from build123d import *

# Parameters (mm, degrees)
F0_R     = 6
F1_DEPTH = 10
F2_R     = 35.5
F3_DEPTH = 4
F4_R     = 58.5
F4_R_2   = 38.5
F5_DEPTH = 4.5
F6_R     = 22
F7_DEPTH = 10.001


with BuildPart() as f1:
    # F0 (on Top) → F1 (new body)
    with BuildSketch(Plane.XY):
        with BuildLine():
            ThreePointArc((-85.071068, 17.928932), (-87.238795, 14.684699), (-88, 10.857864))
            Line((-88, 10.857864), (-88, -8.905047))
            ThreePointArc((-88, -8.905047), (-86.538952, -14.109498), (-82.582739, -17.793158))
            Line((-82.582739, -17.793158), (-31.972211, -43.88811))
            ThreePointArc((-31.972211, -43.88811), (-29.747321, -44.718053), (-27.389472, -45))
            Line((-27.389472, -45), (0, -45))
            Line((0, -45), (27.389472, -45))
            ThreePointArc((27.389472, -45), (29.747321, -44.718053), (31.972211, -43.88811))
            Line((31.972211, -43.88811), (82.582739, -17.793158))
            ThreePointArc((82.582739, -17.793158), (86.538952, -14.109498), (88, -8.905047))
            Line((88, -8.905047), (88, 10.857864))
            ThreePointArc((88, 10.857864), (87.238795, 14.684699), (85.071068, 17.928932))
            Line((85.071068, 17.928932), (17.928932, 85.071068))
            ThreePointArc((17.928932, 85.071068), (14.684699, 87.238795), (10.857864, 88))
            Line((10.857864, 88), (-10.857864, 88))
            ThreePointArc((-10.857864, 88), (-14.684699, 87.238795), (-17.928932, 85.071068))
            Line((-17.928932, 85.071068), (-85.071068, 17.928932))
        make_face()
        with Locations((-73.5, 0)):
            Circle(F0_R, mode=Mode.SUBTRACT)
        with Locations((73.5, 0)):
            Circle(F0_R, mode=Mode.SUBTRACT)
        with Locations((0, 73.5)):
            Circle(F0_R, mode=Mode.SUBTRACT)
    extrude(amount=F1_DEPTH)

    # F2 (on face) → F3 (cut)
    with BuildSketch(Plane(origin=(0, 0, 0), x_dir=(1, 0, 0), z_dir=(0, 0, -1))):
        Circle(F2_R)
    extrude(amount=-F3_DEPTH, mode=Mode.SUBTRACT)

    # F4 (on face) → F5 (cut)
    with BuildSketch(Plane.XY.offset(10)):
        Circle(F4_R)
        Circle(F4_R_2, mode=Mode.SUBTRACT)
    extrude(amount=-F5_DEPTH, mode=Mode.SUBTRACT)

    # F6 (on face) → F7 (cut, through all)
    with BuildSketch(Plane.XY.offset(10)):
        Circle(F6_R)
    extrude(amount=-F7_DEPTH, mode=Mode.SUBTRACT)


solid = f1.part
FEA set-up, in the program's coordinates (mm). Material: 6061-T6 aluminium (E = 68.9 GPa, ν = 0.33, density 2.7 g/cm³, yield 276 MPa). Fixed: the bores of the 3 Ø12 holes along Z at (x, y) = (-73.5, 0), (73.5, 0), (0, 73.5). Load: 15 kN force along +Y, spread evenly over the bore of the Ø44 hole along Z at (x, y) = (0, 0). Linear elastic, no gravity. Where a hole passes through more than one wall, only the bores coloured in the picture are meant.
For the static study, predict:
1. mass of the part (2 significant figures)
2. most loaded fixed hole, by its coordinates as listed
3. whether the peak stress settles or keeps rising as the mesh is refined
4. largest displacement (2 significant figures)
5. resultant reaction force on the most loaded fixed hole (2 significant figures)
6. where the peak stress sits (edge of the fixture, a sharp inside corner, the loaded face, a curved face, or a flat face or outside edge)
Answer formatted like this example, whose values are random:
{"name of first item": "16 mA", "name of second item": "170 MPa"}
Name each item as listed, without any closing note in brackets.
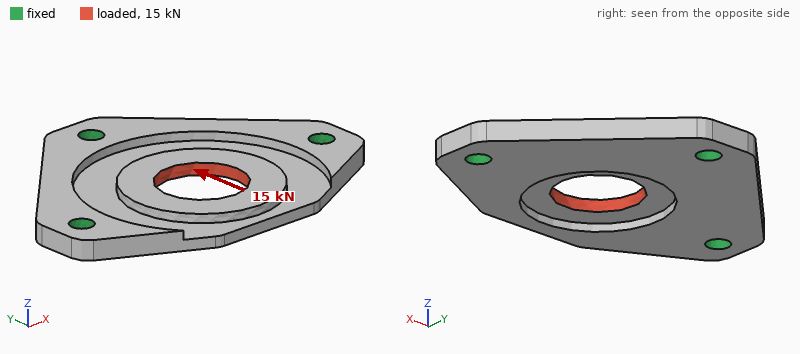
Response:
{"mass of the part": "300 g", "most loaded fixed hole, by its coordinates as listed": "(0, 73.5)", "whether the peak stress settles or keeps rising as the mesh is refined": "keeps rising", "largest displacement": "0.15 mm", "resultant reaction force on the most loaded fixed hole": "6.6 kN", "where the peak stress sits": "a sharp inside corner"}
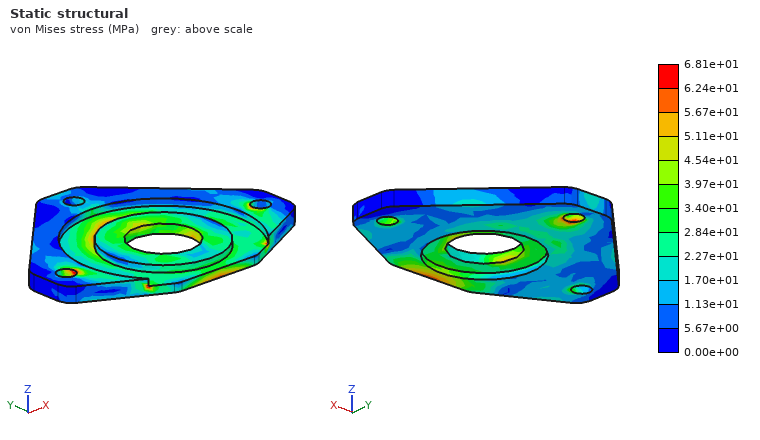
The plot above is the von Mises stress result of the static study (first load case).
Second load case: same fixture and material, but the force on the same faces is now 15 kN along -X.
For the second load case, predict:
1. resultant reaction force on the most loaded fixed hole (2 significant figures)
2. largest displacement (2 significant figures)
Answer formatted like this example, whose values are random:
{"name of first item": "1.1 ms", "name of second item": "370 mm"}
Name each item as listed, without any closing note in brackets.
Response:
{"resultant reaction force on the most loaded fixed hole": "6.2 kN", "largest displacement": "36 µm"}
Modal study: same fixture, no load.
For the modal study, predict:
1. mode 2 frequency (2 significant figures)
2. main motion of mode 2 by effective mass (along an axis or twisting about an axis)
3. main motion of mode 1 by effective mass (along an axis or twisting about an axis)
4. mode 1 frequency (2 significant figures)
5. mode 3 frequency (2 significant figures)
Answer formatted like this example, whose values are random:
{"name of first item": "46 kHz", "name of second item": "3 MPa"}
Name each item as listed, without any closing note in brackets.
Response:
{"mode 2 frequency": "4200 Hz", "main motion of mode 2 by effective mass": "along Z", "main motion of mode 1 by effective mass": "along Z", "mode 1 frequency": "2000 Hz", "mode 3 frequency": "4500 Hz"}
